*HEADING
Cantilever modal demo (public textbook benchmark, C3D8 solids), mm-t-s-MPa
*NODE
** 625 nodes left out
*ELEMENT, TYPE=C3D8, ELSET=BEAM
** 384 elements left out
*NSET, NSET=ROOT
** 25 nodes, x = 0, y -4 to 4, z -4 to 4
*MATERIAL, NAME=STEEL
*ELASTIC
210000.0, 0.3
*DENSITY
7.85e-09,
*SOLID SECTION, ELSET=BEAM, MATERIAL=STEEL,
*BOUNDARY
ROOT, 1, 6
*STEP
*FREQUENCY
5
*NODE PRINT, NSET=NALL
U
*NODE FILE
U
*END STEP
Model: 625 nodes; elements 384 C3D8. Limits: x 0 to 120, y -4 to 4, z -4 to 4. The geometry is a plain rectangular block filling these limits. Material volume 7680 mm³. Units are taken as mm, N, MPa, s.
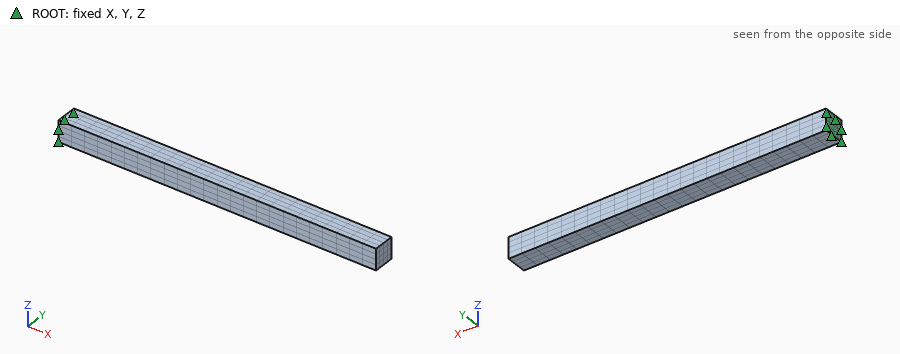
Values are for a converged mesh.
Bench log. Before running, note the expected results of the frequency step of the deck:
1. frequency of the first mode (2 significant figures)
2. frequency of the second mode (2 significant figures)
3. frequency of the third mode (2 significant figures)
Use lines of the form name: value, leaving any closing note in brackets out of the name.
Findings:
frequency of the first mode: 460 Hz
frequency of the second mode: 460 Hz
frequency of the third mode: 2900 Hz
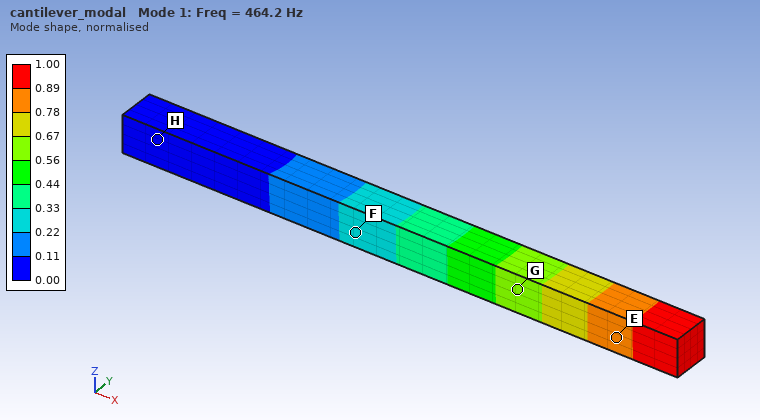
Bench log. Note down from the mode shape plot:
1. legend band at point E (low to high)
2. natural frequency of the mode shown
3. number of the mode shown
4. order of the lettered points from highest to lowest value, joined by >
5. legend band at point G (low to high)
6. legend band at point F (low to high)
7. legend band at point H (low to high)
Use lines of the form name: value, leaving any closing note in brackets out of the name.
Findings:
legend band at point E: 0.78 to 0.89
natural frequency of the mode shown: 464.2 Hz
number of the mode shown: 1
order of the lettered points from highest to lowest value, joined by >: E > G > F > H
legend band at point G: 0.56 to 0.67
legend band at point F: 0.22 to 0.33
legend band at point H: 0.00 to 0.11
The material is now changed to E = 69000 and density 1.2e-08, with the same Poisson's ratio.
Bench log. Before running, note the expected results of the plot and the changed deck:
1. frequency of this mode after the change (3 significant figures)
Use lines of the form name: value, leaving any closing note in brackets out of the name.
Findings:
frequency of this mode after the change: 215 Hz
